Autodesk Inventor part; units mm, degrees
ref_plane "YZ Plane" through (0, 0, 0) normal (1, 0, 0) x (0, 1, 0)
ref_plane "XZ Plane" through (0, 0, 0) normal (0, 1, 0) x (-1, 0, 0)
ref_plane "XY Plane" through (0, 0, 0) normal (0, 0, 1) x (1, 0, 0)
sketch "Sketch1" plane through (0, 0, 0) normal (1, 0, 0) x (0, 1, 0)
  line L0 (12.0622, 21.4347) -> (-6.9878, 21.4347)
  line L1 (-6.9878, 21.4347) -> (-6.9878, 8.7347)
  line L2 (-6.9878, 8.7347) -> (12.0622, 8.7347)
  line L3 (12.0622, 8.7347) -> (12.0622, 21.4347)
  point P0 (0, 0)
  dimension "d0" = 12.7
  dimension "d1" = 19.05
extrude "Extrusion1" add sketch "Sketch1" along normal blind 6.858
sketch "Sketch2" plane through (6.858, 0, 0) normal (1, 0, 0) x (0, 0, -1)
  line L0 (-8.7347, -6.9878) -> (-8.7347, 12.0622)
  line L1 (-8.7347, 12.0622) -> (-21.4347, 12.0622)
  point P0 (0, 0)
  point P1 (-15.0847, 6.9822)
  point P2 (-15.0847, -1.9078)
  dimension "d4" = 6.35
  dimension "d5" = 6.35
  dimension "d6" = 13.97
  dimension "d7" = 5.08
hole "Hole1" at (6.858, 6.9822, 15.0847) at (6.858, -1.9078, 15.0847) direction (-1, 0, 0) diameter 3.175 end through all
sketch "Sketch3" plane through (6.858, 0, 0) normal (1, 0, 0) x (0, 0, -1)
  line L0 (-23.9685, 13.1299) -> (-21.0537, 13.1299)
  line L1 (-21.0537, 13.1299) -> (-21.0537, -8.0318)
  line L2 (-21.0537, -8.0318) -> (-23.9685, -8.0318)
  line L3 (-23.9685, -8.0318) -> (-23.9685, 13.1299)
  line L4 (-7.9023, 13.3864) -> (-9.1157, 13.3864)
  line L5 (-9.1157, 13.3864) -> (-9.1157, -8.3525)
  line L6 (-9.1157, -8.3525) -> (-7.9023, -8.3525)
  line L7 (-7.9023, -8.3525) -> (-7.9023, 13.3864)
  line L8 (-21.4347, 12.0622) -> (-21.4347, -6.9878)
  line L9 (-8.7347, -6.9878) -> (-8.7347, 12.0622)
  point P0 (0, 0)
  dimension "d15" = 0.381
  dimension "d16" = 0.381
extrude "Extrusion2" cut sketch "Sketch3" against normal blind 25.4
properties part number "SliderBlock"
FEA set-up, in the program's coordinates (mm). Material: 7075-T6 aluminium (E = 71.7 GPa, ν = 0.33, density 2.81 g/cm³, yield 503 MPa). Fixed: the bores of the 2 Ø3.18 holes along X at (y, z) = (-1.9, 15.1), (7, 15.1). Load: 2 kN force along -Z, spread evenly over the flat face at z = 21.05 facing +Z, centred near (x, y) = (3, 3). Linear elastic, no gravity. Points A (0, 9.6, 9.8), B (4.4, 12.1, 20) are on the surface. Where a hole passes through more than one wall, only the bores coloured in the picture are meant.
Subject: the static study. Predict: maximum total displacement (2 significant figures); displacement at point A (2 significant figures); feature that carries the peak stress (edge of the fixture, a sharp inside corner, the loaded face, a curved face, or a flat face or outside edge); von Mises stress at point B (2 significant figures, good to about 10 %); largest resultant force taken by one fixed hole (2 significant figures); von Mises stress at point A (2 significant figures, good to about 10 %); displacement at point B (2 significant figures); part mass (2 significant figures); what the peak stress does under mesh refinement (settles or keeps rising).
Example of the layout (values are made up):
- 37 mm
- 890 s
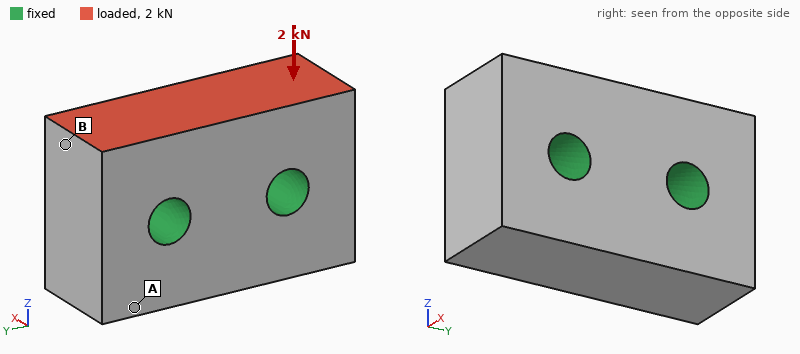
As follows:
- 2.3 µm
- 0.50 µm
- edge of the fixture
- 15 MPa
- 1.0 kN
- 3.0 MPa
- 2.0 µm
- 4.1 g
- keeps rising
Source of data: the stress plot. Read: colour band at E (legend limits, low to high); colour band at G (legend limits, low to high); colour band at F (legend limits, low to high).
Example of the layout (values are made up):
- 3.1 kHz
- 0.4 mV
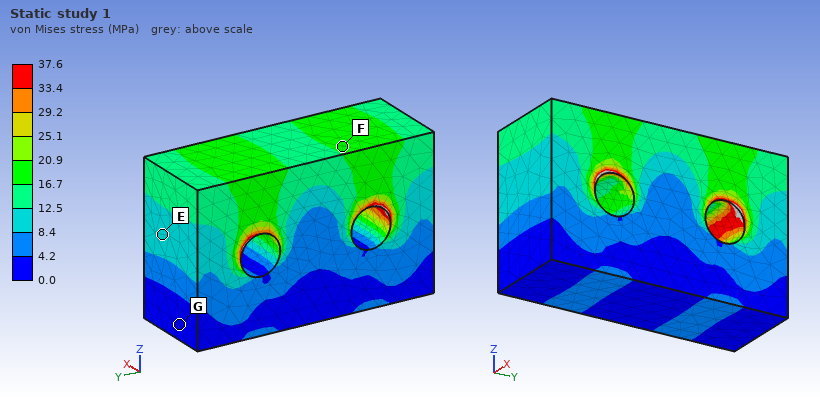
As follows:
- 8.4 to 12.5 MPa
- 0.0 to 4.2 MPa
- 16.7 to 20.9 MPa
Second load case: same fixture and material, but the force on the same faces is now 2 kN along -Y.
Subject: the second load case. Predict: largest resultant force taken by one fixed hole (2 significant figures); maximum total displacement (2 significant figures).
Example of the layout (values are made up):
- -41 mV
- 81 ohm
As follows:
- 1.3 kN
- 7.6 µm
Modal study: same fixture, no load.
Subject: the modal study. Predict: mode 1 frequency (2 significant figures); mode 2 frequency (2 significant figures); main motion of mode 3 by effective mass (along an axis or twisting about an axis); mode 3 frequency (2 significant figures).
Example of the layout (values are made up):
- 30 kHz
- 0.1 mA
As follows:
- 91 kHz
- 94 kHz
- twisting about Z
- 100 kHz
